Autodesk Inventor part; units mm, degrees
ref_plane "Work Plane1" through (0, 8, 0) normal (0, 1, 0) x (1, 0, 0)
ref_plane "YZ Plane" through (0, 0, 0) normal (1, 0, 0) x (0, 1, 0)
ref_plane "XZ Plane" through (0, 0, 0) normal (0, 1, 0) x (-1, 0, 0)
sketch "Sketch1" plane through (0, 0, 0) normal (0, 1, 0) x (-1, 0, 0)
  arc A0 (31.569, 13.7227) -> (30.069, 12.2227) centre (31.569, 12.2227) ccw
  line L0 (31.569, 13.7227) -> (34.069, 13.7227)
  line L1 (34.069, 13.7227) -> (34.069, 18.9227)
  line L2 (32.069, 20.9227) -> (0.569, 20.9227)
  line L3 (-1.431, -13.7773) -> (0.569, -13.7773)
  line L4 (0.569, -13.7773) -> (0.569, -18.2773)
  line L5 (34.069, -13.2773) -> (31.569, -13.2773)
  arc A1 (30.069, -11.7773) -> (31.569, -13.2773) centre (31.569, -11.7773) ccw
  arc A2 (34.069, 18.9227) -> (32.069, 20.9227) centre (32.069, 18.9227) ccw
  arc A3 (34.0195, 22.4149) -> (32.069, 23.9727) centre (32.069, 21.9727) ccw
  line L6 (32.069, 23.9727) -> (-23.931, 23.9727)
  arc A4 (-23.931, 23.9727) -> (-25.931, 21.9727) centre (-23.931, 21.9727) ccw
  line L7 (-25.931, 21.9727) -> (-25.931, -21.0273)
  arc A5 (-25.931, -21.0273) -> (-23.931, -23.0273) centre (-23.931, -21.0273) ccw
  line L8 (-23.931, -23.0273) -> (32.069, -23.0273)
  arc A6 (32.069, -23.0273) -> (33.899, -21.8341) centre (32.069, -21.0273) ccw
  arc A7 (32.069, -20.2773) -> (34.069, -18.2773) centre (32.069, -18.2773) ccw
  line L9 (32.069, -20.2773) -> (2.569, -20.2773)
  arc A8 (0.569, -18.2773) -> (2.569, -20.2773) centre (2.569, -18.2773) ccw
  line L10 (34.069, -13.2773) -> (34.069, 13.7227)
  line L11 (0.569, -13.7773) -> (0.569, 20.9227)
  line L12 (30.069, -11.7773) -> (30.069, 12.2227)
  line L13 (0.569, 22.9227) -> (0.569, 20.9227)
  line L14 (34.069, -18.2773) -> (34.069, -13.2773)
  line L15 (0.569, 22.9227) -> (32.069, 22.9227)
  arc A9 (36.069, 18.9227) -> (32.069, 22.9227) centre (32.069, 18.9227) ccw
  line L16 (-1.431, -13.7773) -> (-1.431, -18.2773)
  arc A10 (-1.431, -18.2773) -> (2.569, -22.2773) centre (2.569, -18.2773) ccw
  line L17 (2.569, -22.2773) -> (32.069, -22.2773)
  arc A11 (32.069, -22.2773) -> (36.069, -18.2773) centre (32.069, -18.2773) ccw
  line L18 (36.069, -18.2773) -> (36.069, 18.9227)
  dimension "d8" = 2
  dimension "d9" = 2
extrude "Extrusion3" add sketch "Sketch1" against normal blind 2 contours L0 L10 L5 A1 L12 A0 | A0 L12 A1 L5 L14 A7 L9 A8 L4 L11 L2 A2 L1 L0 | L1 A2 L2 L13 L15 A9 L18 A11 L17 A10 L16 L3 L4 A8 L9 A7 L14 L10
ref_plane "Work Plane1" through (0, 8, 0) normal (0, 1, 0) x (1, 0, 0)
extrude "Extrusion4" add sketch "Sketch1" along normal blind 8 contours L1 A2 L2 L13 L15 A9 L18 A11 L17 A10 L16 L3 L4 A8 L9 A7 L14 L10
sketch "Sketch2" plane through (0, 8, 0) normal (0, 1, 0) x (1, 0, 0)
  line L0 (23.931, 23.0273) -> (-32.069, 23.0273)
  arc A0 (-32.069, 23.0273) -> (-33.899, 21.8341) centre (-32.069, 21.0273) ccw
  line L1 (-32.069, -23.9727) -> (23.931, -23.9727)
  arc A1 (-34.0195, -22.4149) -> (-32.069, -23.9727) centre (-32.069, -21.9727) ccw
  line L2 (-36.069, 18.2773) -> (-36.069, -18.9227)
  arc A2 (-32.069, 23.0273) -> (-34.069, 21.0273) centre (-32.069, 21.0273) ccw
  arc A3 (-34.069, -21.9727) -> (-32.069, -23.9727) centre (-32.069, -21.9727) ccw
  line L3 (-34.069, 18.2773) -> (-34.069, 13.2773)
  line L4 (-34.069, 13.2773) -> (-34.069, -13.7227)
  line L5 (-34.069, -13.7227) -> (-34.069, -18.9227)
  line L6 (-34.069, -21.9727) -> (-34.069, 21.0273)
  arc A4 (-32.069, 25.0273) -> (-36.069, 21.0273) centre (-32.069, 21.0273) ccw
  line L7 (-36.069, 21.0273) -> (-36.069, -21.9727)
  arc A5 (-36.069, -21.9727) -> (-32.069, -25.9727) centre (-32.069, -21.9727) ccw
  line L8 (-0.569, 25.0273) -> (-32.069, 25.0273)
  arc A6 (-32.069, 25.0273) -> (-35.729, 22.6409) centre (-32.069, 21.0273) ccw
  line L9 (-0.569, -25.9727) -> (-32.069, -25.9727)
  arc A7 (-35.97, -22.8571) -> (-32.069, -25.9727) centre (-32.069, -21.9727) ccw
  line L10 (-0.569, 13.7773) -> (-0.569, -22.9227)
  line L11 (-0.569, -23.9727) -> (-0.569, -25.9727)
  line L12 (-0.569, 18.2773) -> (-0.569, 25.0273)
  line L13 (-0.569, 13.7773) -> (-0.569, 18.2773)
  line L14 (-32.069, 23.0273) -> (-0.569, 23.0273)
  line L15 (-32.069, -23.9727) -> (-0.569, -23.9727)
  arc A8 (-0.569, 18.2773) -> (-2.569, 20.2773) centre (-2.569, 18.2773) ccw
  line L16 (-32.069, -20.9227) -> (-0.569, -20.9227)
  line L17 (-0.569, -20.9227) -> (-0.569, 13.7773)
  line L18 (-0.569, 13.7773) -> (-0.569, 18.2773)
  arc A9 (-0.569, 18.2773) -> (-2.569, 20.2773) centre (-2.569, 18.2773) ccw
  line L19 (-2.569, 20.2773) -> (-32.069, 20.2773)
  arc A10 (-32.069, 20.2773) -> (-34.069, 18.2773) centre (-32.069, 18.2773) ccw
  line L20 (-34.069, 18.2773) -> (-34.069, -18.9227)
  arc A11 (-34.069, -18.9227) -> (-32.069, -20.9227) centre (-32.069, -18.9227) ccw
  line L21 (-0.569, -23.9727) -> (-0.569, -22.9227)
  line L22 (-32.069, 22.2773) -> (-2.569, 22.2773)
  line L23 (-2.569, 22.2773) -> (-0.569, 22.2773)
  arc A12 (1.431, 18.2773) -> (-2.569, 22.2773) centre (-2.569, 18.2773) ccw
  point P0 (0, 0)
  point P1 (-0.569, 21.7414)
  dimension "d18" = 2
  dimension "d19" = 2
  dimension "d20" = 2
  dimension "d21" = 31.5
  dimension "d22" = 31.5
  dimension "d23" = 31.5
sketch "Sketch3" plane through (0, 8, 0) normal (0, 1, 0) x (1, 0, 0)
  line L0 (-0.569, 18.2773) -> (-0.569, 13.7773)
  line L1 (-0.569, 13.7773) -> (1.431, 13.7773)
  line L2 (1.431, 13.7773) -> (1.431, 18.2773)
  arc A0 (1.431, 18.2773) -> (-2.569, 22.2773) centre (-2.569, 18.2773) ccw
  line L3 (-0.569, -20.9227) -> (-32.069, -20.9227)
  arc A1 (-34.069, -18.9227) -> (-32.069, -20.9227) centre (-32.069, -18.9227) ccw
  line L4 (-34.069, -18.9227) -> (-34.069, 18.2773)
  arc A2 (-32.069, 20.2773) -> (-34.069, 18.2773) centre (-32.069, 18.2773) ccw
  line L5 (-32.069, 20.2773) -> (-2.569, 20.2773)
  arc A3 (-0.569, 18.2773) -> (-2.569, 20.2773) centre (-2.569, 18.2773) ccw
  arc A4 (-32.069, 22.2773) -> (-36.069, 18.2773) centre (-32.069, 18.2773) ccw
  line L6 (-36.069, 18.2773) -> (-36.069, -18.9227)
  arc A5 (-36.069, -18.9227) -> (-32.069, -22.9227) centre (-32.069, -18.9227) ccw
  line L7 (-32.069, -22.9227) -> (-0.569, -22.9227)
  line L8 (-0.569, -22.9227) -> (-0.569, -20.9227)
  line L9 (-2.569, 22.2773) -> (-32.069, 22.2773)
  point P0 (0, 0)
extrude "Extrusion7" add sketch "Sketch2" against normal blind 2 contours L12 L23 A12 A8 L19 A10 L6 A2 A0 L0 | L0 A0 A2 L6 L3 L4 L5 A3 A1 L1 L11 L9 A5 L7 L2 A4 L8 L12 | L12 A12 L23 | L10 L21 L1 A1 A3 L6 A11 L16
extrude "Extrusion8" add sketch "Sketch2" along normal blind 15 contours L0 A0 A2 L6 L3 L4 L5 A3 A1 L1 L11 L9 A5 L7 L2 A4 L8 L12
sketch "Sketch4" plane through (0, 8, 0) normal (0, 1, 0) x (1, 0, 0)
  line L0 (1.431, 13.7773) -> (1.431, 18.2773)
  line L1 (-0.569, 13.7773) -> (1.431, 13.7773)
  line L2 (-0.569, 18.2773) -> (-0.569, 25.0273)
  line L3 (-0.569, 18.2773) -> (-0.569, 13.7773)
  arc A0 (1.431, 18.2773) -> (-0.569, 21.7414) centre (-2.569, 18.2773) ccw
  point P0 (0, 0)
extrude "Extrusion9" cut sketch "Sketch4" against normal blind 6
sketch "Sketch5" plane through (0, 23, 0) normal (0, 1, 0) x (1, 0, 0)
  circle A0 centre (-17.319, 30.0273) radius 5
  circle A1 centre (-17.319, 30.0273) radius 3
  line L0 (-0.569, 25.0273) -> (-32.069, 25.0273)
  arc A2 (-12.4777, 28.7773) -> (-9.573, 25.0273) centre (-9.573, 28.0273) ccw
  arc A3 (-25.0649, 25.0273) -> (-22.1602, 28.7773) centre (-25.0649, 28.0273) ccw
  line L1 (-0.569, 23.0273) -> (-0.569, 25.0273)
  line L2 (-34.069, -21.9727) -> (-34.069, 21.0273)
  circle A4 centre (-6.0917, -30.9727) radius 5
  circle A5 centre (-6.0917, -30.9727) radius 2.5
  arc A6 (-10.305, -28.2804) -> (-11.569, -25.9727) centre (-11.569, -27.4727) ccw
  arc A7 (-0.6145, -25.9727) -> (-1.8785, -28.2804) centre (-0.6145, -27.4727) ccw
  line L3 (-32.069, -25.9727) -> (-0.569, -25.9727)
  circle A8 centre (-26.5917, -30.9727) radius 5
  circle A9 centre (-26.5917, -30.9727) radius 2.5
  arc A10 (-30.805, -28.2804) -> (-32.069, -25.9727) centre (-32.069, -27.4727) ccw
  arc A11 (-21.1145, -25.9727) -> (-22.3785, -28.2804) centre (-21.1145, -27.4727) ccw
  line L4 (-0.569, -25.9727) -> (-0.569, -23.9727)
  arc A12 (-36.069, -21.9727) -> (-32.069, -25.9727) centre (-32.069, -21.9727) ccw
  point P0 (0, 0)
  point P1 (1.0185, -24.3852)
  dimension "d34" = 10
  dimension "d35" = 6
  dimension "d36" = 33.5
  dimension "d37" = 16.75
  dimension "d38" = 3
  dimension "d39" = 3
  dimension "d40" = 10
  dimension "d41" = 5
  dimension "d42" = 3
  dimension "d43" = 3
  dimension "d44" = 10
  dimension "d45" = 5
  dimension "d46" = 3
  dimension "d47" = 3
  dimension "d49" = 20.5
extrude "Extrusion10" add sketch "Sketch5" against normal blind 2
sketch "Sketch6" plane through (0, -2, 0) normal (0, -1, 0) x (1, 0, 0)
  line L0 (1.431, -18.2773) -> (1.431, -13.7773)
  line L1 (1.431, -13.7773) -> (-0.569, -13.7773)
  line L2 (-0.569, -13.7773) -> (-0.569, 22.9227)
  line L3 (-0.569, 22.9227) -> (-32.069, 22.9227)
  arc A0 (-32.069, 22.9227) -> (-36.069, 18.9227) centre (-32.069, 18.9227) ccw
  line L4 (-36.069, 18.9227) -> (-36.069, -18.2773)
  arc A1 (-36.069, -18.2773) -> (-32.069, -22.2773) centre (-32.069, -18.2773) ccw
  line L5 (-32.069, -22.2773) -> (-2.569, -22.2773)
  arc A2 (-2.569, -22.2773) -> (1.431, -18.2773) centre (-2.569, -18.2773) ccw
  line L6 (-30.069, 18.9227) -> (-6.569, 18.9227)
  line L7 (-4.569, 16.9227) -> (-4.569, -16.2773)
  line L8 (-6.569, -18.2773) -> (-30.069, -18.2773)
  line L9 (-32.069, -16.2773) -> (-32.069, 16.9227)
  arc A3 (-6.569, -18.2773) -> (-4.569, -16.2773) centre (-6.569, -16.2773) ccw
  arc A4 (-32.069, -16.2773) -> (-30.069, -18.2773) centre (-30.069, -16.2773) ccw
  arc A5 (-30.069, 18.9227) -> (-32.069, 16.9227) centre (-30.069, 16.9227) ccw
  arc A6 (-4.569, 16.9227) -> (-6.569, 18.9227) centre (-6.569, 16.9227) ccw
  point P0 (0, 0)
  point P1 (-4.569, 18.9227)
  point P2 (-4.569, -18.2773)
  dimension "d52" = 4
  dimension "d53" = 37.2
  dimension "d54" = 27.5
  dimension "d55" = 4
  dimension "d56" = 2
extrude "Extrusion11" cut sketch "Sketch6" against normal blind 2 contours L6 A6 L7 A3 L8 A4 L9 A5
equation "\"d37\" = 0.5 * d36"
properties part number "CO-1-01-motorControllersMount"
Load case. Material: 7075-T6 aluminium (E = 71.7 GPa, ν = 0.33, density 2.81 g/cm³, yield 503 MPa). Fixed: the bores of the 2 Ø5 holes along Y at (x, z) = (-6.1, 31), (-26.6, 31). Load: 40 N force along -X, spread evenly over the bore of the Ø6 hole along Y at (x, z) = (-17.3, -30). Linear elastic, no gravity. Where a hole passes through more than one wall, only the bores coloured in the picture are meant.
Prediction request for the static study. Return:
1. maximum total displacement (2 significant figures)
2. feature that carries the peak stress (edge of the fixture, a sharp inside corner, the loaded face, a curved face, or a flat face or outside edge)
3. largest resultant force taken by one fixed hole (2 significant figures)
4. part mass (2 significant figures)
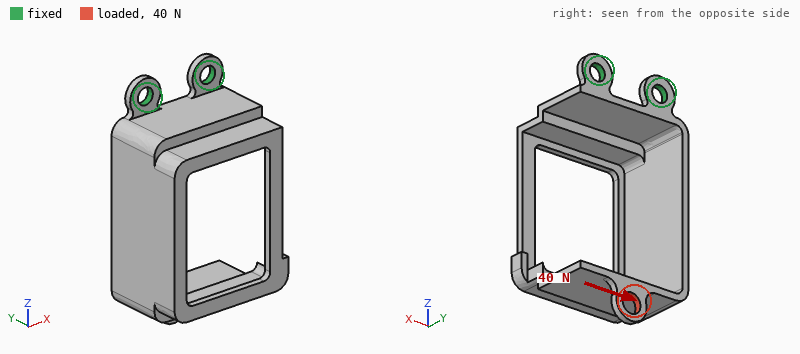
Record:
0.99 mm
a curved face
78 N
20 g
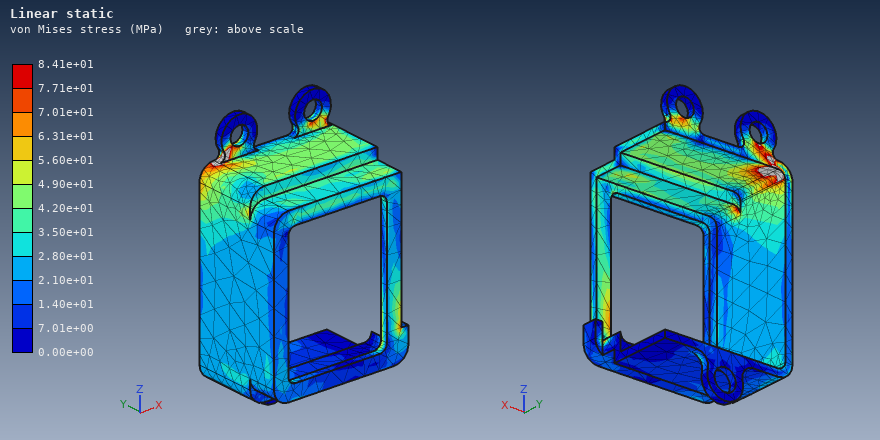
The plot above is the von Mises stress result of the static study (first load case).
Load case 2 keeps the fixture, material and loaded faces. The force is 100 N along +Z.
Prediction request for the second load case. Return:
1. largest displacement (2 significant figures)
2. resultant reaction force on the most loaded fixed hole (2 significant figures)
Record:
0.88 mm
55 N
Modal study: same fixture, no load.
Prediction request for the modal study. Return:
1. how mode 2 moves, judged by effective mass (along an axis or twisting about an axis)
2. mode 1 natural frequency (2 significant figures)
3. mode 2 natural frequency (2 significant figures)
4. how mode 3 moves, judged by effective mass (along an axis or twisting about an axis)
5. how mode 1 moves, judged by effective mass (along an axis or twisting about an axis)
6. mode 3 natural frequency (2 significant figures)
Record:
along X
300 Hz
480 Hz
along Z
along Y
1100 Hz
